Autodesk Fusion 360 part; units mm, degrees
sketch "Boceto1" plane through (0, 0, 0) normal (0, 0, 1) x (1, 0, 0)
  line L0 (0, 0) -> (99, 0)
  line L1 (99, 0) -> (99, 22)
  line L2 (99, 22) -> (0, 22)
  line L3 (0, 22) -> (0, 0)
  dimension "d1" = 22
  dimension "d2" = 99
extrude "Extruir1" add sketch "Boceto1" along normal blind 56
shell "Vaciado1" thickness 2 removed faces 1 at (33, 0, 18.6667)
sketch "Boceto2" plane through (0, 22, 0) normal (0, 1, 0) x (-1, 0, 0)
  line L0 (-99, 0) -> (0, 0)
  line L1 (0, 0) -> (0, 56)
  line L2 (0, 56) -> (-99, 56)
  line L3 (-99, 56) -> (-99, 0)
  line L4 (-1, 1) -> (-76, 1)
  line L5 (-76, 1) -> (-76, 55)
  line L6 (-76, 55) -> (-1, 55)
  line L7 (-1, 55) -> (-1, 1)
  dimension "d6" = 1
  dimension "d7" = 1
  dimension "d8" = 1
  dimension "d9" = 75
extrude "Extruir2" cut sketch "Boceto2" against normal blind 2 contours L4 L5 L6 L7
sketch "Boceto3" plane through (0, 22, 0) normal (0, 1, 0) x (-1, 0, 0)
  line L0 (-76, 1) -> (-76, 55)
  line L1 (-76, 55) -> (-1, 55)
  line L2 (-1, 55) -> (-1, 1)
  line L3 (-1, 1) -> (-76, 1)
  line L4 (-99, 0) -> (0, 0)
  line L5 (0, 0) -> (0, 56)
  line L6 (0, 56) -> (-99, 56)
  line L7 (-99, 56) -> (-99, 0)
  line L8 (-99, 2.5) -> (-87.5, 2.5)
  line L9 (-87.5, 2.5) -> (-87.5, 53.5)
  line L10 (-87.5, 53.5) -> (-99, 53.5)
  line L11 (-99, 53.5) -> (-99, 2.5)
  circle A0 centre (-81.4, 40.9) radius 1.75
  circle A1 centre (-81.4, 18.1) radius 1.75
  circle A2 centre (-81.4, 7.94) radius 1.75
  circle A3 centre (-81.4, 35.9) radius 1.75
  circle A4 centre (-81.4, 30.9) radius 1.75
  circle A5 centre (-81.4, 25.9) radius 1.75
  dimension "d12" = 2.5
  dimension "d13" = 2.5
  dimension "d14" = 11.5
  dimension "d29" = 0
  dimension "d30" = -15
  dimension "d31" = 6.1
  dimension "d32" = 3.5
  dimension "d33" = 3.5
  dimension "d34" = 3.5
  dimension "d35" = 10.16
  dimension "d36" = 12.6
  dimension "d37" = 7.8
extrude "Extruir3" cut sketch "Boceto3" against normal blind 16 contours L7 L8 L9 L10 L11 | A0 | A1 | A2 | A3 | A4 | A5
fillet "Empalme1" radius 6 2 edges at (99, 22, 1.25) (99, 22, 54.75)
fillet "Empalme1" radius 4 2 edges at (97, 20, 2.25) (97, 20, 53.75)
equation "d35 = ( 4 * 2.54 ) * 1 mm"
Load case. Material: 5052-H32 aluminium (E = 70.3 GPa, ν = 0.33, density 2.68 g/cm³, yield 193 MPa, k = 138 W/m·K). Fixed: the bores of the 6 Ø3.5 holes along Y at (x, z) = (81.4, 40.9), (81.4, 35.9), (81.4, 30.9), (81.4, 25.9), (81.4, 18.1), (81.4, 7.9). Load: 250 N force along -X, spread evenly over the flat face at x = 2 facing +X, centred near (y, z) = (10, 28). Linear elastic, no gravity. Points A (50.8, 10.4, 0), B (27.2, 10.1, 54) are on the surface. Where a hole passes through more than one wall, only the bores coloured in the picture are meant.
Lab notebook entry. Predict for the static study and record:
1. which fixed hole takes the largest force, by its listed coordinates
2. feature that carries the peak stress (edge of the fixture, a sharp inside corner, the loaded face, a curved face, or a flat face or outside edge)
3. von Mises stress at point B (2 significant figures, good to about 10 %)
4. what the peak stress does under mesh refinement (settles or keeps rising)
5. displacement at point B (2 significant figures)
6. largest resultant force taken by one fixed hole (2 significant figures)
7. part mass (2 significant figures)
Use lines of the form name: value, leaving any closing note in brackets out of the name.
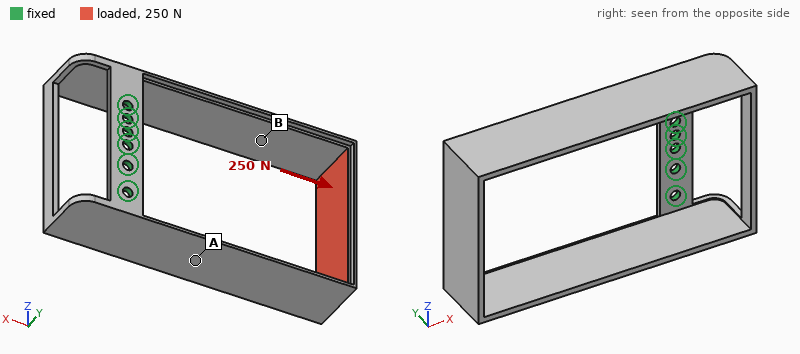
which fixed hole takes the largest force, by its listed coordinates: (81.4, 40.9)
feature that carries the peak stress: edge of the fixture
von Mises stress at point B: 29 MPa
what the peak stress does under mesh refinement: keeps rising
displacement at point B: 0.73 mm
largest resultant force taken by one fixed hole: 260 N
part mass: 33 g
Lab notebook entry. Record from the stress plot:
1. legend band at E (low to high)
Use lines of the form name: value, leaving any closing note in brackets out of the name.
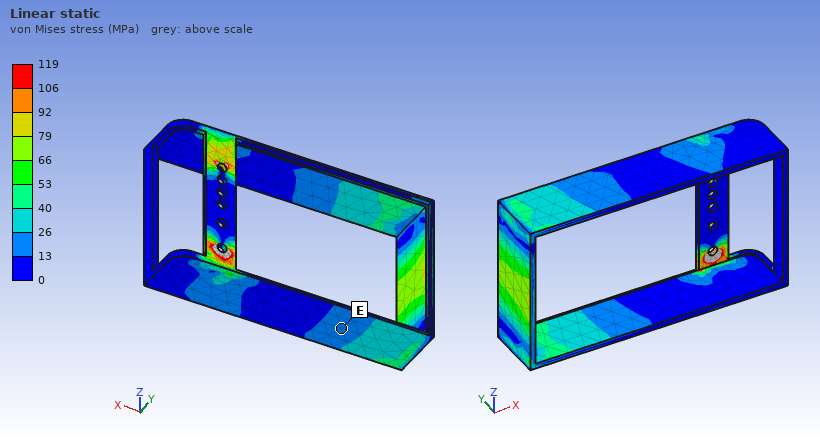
legend band at E: 13 to 26 MPa
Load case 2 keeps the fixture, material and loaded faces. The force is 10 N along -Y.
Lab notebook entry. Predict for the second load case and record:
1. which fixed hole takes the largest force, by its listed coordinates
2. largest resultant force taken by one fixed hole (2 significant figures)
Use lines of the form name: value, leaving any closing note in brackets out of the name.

which fixed hole takes the largest force, by its listed coordinates: (81.4, 40.9)
largest resultant force taken by one fixed hole: 6.9 N
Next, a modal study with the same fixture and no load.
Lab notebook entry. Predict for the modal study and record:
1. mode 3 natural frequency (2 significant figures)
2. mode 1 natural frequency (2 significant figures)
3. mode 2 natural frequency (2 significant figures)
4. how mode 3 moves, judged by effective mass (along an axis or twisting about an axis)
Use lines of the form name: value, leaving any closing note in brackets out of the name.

mode 3 natural frequency: 560 Hz
mode 1 natural frequency: 260 Hz
mode 2 natural frequency: 260 Hz
how mode 3 moves, judged by effective mass: twisting about X
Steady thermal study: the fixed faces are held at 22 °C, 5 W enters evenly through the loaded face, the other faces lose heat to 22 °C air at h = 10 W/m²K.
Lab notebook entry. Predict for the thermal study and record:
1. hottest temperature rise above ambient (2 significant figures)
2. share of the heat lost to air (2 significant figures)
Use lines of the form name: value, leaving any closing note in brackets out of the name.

hottest temperature rise above ambient: 36 K
share of the heat lost to air: 41 %
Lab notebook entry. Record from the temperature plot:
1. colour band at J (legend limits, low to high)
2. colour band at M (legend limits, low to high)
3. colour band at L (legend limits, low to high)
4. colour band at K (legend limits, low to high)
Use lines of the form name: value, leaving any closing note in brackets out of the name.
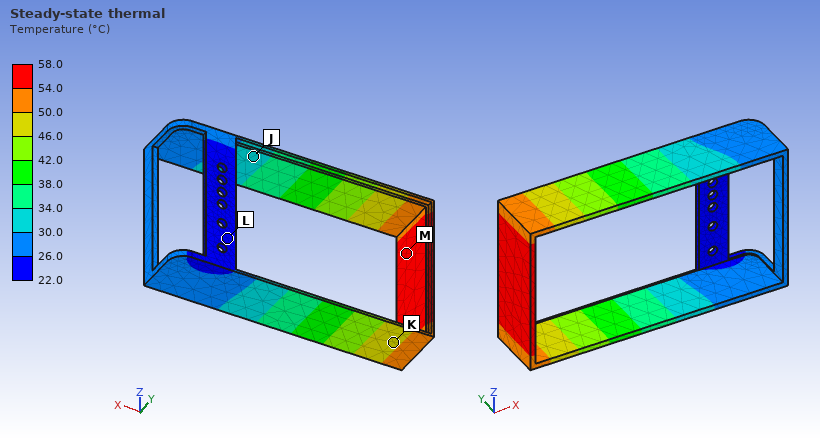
colour band at J: 30.0 to 34.0 °C
colour band at M: 54.0 to 58.0 °C
colour band at L: 22.0 to 26.0 °C
colour band at K: 46.0 to 50.0 °C
